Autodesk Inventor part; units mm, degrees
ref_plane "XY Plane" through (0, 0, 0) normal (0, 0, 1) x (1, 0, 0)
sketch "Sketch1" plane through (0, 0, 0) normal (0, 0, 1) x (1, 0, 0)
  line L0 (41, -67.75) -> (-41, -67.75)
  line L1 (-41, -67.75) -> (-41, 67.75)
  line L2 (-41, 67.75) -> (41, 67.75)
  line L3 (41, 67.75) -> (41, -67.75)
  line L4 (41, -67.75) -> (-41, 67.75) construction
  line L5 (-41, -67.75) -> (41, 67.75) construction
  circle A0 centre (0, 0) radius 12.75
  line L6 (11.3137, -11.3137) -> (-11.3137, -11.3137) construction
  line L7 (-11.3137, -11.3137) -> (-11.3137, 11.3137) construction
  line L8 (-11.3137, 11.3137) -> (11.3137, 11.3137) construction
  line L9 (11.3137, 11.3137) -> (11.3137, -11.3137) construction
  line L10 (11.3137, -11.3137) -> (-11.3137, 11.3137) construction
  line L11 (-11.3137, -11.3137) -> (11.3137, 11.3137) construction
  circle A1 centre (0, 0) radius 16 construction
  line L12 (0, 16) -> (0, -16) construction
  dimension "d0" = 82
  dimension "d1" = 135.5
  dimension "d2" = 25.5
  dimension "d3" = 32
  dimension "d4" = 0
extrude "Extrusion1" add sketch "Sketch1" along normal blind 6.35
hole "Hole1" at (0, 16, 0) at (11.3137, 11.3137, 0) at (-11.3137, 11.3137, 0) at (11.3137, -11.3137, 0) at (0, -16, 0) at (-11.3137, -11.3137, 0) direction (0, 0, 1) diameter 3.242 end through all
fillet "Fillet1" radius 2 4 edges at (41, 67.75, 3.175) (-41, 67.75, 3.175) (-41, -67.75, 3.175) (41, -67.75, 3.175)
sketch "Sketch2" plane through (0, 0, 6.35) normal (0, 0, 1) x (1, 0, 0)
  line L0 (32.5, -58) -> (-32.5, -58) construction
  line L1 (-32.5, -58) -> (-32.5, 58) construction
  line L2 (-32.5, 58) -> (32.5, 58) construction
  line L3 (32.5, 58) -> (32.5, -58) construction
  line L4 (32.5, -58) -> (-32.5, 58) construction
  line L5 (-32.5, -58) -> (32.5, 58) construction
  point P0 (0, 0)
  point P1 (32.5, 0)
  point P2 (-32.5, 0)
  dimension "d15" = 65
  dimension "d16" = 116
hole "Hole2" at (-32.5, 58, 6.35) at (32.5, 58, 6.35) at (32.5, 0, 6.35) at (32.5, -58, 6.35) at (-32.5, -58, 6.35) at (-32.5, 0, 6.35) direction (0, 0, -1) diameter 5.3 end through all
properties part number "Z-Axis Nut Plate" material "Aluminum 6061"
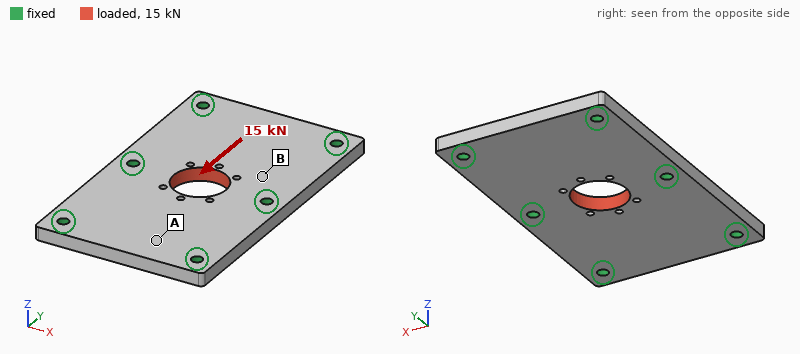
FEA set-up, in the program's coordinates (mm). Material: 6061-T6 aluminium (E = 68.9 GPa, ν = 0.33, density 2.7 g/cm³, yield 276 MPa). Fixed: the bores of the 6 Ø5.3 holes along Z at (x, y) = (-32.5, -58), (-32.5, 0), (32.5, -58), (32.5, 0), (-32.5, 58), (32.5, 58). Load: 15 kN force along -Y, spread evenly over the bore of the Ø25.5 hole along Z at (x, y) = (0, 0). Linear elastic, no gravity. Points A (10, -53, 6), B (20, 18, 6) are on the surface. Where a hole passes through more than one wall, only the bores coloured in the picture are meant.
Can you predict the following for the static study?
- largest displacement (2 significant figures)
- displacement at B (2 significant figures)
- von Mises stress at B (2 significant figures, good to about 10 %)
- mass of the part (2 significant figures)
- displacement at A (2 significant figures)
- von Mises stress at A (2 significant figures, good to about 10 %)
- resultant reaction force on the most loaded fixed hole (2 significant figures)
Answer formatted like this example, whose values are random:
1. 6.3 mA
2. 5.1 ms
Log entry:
1. 19 µm
2. 8.3 µm
3. 21 MPa
4. 180 g
5. 6.6 µm
6. 6.8 MPa
7. 3.6 kN
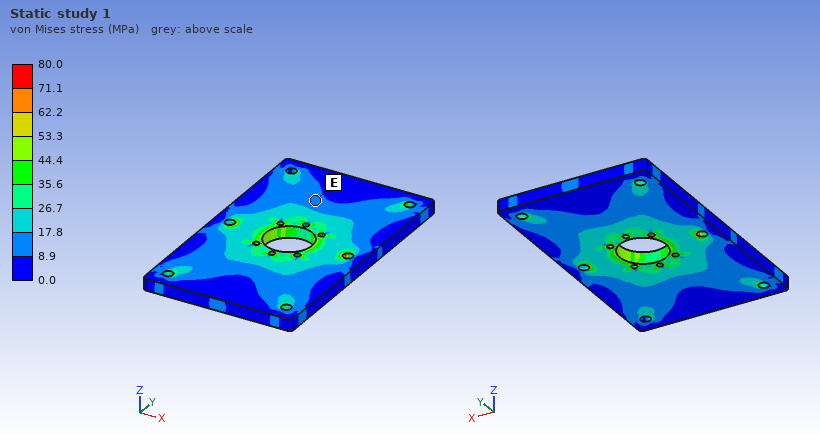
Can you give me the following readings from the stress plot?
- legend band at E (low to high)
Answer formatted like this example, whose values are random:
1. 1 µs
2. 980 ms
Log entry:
1. 8.9 to 17.8 MPa
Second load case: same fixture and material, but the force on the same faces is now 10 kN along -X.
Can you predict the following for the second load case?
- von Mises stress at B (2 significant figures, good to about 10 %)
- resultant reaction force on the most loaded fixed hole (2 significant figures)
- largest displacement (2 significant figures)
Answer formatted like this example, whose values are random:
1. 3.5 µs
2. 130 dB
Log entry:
1. 7.2 MPa
2. 3.6 kN
3. 11 µm
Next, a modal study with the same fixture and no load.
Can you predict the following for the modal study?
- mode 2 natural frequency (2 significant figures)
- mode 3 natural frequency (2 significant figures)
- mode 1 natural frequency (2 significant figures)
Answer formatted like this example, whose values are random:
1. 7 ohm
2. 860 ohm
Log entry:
1. 5900 Hz
2. 8800 Hz
3. 5700 Hz
